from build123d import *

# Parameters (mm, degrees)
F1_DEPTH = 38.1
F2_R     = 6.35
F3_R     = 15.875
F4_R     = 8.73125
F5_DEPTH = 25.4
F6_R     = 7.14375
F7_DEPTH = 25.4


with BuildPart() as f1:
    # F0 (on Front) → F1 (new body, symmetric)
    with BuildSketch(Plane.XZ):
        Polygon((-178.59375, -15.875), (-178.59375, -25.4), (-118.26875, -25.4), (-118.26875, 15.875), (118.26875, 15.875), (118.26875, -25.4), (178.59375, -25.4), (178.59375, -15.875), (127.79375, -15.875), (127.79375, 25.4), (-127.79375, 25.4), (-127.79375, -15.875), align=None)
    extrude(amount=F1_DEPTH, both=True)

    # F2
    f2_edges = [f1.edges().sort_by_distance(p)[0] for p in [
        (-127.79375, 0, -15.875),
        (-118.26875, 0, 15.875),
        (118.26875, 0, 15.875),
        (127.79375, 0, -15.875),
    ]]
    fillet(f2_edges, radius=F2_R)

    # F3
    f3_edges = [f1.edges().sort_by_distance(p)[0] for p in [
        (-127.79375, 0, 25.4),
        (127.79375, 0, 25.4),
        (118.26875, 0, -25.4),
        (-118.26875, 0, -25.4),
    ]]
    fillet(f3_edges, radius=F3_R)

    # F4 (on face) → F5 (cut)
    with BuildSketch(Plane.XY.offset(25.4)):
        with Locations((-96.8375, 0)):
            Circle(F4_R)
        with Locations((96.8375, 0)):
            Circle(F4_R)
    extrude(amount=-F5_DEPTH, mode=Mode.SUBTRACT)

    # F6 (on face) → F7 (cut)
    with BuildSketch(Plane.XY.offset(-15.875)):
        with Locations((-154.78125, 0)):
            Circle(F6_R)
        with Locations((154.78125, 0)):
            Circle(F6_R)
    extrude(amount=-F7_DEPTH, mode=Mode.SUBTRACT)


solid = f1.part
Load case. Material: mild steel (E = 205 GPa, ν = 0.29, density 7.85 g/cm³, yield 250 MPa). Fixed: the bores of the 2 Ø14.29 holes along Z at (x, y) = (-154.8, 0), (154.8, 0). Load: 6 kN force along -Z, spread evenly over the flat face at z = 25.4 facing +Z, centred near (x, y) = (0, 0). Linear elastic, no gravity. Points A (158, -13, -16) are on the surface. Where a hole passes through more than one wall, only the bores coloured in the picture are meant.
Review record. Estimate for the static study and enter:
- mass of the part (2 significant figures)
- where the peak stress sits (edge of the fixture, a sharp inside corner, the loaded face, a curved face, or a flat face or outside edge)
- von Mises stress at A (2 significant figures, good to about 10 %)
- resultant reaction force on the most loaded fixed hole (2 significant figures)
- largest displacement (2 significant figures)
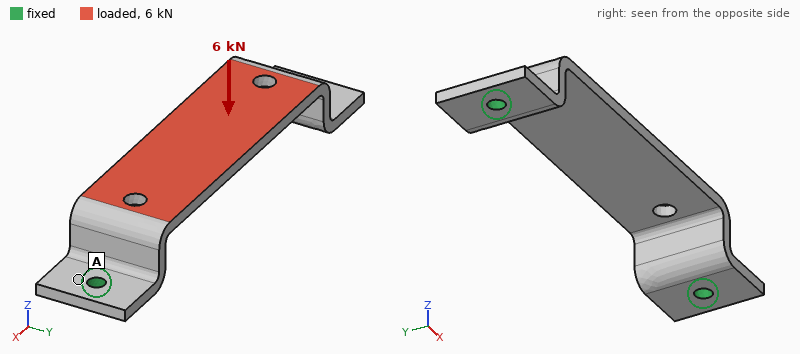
2.3 kg
a curved face
8.7 MPa
5.4 kN
0.30 mm
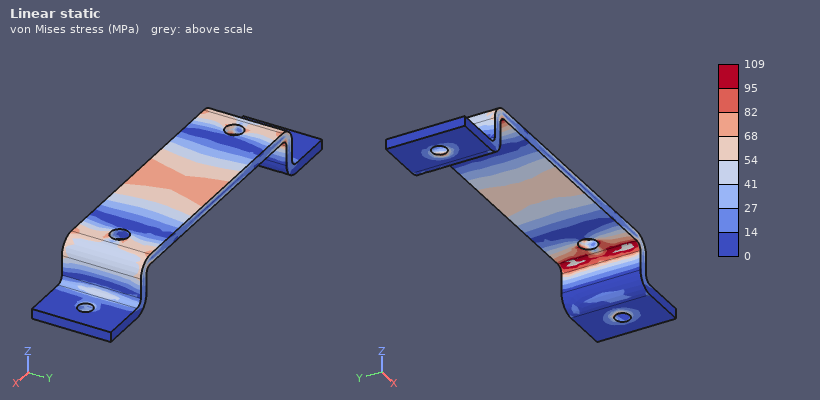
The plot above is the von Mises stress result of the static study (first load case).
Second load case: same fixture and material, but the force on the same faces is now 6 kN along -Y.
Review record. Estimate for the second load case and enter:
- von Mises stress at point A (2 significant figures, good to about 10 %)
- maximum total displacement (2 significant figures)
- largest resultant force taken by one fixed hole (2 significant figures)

59 MPa
0.14 mm
3.0 kN
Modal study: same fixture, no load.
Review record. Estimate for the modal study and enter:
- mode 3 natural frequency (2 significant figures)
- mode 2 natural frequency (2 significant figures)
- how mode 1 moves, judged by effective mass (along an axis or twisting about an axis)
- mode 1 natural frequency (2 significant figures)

960 Hz
940 Hz
along Z
740 Hz
